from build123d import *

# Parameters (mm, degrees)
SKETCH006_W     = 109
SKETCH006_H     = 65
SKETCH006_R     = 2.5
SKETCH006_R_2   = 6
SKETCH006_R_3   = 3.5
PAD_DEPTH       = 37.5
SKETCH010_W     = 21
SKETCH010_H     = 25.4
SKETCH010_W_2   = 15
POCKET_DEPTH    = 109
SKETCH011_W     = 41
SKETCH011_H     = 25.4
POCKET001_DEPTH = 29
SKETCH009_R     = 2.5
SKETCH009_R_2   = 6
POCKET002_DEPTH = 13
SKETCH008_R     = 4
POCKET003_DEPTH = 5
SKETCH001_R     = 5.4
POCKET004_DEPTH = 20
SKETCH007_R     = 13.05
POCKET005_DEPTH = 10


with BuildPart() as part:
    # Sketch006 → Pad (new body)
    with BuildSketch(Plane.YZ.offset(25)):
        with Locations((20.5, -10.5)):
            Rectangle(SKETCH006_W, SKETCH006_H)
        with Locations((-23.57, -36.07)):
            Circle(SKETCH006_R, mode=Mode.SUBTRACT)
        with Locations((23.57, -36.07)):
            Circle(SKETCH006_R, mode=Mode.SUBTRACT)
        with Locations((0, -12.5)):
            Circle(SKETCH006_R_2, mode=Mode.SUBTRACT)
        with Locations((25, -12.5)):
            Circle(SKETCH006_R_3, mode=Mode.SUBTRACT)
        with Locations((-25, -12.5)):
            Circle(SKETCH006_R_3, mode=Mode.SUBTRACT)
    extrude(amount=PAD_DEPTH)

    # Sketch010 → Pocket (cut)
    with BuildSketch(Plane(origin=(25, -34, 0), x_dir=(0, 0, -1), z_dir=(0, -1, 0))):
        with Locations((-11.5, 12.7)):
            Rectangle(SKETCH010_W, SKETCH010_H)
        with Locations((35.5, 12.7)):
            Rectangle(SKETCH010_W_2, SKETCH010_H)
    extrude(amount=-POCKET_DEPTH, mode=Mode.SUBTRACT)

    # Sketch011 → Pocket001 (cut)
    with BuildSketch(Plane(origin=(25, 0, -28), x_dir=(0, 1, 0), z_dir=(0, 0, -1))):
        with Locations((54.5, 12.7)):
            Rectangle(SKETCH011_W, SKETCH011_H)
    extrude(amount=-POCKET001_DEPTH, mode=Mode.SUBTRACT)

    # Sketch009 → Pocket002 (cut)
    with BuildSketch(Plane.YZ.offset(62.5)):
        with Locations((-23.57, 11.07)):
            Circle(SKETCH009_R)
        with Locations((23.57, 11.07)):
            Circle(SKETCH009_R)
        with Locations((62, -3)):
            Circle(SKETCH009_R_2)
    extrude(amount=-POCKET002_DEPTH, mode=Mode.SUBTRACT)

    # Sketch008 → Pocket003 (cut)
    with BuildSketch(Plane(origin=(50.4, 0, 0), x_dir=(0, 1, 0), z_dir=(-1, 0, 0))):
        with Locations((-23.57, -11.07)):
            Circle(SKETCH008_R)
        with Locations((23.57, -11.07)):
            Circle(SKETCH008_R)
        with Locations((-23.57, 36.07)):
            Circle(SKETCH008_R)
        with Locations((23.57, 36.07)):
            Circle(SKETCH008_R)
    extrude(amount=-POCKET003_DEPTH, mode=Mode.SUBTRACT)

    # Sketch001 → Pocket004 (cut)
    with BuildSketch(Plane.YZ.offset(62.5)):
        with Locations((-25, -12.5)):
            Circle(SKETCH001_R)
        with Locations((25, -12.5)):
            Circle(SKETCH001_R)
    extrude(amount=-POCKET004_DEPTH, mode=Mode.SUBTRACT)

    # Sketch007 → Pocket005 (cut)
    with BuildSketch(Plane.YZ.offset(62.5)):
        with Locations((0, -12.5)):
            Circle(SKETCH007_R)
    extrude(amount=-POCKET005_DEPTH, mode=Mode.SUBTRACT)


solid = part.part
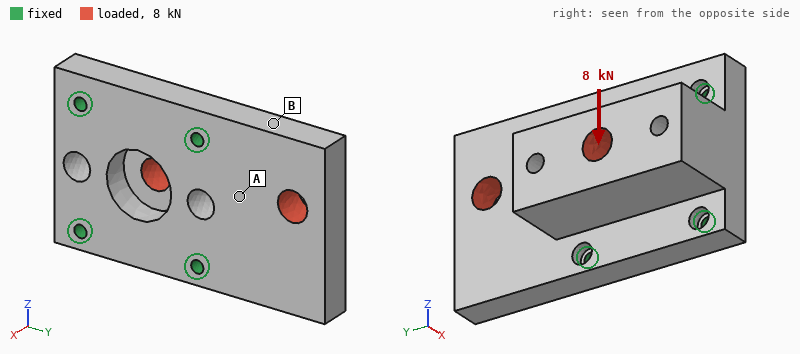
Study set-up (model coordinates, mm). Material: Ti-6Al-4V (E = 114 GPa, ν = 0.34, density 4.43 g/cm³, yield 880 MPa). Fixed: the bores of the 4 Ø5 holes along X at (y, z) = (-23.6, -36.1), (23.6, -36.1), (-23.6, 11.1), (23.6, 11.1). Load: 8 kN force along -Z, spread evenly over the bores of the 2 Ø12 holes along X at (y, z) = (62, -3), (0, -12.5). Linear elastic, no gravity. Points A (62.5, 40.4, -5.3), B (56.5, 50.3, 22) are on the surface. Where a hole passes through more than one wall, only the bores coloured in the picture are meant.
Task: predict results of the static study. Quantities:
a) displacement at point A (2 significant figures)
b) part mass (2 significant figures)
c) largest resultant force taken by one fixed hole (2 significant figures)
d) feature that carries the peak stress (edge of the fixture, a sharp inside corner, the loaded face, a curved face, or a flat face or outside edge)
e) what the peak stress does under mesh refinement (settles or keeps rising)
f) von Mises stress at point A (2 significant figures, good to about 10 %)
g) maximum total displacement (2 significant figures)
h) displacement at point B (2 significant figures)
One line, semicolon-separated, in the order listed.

2.9 µm; 530 g; 3.2 kN; edge of the fixture; keeps rising; 9.9 MPa; 8.7 µm; 5.5 µm
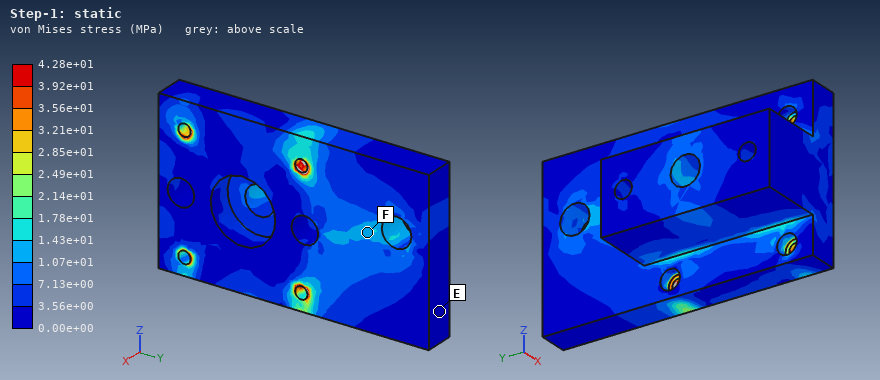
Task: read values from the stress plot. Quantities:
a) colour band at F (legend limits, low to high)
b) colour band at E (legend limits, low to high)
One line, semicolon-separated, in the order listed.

1.07e+01 to 1.43e+01 MPa; 0.00e+00 to 3.56e+00 MPa
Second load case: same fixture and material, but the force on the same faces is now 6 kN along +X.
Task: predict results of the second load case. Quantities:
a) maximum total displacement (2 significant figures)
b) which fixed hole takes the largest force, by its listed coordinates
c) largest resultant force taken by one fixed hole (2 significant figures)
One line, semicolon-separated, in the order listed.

68 µm; (23.6, 11.1); 3.2 kN
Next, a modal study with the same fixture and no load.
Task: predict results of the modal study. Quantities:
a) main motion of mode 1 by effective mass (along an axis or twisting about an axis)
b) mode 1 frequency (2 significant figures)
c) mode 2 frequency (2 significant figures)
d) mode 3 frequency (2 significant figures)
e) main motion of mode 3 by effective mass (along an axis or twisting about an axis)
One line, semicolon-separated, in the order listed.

along X; 3400 Hz; 6300 Hz; 9600 Hz; along Z
